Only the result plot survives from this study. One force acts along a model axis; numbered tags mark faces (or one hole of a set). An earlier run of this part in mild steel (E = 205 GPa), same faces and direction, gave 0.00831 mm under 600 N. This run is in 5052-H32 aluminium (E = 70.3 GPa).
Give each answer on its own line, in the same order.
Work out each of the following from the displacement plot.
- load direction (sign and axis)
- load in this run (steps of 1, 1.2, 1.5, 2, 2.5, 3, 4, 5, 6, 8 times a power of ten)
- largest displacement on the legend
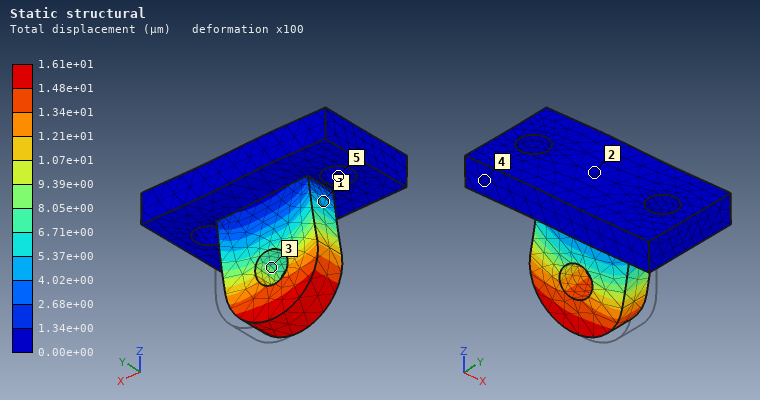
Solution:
-X
400 N
1.61e+01 µm
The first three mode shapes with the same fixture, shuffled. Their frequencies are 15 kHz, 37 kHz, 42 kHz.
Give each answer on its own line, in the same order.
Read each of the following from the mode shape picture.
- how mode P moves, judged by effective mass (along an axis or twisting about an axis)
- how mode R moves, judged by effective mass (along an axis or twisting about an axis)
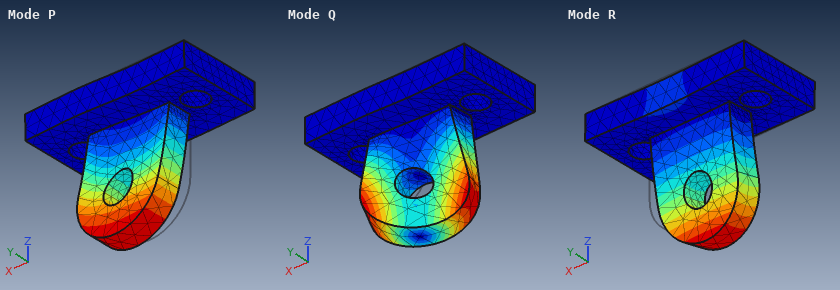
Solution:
along X
along Y
